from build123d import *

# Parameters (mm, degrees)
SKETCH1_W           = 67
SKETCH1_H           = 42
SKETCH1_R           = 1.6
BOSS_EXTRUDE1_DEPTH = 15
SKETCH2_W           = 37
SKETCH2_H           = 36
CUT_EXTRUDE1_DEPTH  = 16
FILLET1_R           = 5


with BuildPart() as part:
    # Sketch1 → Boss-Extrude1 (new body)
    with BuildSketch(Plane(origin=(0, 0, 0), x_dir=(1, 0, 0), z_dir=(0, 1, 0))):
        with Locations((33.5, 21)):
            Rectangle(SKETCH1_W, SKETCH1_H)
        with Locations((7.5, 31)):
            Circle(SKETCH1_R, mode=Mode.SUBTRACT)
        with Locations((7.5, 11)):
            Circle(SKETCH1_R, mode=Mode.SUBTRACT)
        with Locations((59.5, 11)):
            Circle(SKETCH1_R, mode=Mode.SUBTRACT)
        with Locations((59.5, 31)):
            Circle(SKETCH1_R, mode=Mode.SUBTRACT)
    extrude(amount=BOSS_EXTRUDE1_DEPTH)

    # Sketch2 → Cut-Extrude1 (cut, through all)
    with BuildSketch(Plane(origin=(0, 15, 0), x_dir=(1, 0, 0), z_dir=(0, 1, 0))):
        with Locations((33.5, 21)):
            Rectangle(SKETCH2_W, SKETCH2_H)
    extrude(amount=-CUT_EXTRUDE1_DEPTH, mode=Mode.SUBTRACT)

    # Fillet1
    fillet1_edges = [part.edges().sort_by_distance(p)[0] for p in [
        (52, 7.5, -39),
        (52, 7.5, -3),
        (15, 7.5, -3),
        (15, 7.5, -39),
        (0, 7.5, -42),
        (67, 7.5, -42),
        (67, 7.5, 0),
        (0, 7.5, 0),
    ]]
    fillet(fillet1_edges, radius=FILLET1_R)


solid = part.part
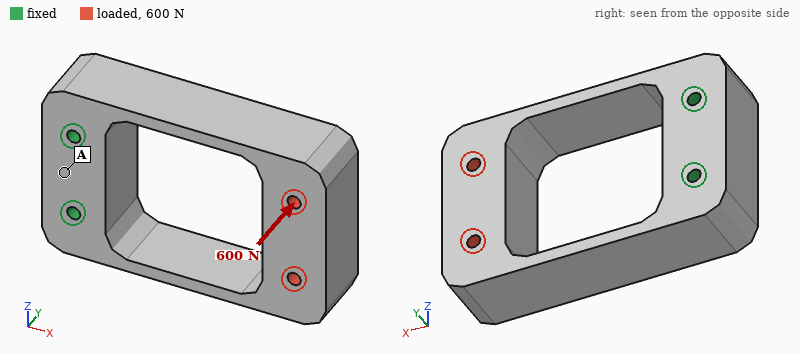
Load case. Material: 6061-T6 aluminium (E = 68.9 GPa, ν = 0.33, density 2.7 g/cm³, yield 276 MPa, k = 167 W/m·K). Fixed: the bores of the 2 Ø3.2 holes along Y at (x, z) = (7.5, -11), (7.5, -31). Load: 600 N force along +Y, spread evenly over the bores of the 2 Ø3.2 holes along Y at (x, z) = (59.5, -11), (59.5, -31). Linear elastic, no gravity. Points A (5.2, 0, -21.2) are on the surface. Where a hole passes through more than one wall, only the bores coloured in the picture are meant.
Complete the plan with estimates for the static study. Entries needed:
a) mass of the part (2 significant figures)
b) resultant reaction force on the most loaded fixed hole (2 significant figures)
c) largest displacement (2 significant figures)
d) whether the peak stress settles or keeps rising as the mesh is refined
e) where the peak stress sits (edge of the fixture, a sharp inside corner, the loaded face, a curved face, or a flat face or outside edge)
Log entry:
59 g
300 N
0.28 mm
keeps rising
a sharp inside corner
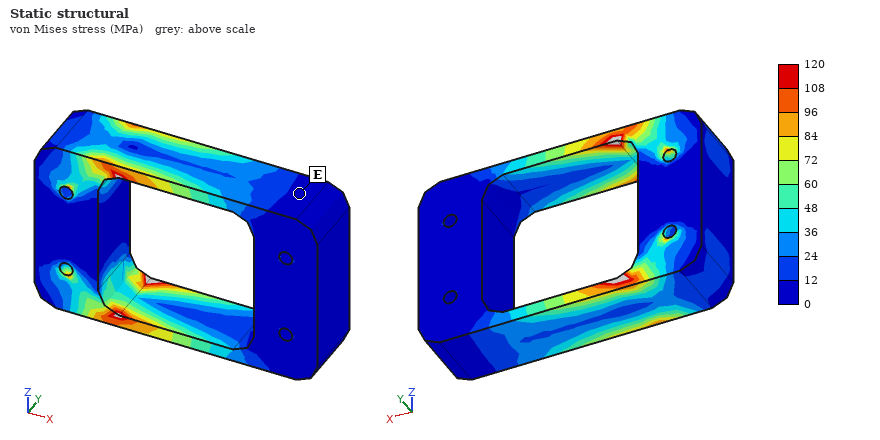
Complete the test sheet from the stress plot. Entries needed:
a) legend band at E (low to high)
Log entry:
0 to 12 MPa
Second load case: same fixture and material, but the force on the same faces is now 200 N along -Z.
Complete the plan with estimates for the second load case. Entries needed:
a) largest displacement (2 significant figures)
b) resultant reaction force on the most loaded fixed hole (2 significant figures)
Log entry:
0.15 mm
420 N
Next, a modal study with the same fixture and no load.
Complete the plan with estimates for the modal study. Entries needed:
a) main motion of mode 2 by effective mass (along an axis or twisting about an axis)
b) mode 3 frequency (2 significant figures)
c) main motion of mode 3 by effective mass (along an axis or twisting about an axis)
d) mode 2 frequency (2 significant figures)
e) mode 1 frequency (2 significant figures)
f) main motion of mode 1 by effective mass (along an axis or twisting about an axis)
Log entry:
along Y
4200 Hz
twisting about X
1600 Hz
1100 Hz
along Z
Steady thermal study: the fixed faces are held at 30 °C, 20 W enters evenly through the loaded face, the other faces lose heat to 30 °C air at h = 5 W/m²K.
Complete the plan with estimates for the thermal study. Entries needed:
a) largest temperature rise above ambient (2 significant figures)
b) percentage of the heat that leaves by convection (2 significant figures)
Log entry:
54 K
5.4 %
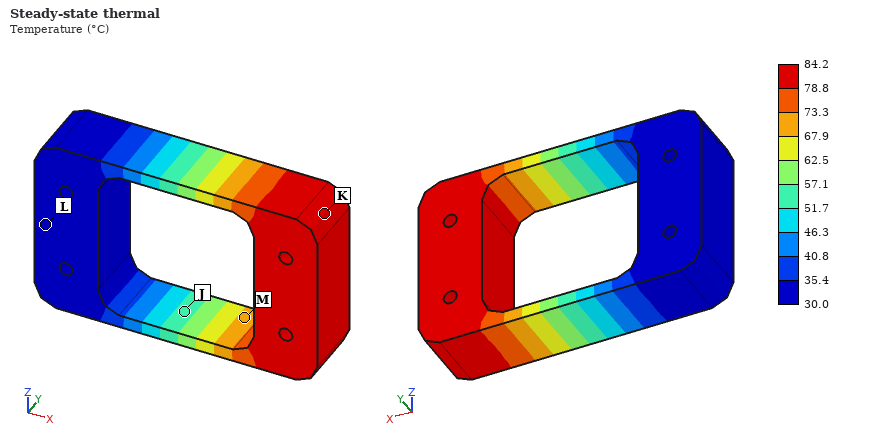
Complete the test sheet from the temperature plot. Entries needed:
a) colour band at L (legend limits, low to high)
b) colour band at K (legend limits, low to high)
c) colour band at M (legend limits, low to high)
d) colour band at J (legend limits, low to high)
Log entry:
30.0 to 35.4 °C
78.8 to 84.2 °C
67.9 to 73.3 °C
51.7 to 57.1 °C
